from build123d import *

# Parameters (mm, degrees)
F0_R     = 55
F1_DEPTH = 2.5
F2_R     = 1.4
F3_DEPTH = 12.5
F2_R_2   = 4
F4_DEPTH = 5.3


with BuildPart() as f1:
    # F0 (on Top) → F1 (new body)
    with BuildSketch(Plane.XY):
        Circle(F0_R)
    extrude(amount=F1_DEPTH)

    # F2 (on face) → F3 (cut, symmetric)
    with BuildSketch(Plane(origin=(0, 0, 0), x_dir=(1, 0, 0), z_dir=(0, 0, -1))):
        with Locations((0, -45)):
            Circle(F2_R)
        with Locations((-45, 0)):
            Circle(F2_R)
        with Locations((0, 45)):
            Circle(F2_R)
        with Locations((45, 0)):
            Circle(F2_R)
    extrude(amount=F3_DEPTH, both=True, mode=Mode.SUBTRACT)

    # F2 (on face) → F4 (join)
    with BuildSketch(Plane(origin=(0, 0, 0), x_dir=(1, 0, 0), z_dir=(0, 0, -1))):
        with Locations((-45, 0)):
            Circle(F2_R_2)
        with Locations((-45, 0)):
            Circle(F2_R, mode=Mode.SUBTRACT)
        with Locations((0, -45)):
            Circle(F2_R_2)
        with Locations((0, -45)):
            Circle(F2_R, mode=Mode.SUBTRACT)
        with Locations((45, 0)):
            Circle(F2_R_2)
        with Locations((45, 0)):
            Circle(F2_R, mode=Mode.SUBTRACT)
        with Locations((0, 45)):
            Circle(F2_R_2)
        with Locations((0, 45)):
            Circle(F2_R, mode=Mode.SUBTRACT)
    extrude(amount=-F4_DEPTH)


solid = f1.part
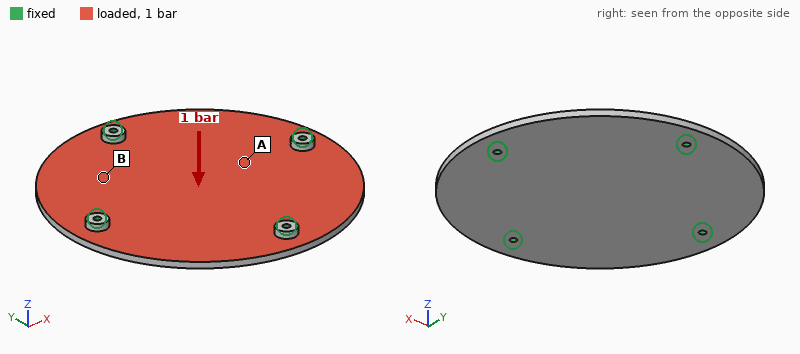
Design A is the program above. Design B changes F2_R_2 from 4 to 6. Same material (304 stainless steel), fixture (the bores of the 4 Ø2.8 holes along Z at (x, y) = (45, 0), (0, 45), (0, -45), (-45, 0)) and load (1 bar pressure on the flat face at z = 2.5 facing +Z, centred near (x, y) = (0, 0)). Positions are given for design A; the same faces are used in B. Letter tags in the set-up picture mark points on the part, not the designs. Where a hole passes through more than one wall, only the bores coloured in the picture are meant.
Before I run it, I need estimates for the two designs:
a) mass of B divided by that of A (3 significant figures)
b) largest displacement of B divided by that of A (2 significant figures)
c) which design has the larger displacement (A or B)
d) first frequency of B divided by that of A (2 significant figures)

1.03
0.83
A
1.1
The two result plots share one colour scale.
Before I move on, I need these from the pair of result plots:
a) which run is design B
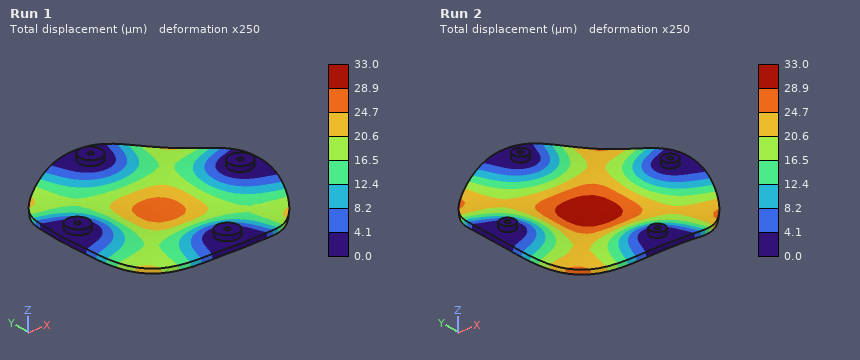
Run 1
